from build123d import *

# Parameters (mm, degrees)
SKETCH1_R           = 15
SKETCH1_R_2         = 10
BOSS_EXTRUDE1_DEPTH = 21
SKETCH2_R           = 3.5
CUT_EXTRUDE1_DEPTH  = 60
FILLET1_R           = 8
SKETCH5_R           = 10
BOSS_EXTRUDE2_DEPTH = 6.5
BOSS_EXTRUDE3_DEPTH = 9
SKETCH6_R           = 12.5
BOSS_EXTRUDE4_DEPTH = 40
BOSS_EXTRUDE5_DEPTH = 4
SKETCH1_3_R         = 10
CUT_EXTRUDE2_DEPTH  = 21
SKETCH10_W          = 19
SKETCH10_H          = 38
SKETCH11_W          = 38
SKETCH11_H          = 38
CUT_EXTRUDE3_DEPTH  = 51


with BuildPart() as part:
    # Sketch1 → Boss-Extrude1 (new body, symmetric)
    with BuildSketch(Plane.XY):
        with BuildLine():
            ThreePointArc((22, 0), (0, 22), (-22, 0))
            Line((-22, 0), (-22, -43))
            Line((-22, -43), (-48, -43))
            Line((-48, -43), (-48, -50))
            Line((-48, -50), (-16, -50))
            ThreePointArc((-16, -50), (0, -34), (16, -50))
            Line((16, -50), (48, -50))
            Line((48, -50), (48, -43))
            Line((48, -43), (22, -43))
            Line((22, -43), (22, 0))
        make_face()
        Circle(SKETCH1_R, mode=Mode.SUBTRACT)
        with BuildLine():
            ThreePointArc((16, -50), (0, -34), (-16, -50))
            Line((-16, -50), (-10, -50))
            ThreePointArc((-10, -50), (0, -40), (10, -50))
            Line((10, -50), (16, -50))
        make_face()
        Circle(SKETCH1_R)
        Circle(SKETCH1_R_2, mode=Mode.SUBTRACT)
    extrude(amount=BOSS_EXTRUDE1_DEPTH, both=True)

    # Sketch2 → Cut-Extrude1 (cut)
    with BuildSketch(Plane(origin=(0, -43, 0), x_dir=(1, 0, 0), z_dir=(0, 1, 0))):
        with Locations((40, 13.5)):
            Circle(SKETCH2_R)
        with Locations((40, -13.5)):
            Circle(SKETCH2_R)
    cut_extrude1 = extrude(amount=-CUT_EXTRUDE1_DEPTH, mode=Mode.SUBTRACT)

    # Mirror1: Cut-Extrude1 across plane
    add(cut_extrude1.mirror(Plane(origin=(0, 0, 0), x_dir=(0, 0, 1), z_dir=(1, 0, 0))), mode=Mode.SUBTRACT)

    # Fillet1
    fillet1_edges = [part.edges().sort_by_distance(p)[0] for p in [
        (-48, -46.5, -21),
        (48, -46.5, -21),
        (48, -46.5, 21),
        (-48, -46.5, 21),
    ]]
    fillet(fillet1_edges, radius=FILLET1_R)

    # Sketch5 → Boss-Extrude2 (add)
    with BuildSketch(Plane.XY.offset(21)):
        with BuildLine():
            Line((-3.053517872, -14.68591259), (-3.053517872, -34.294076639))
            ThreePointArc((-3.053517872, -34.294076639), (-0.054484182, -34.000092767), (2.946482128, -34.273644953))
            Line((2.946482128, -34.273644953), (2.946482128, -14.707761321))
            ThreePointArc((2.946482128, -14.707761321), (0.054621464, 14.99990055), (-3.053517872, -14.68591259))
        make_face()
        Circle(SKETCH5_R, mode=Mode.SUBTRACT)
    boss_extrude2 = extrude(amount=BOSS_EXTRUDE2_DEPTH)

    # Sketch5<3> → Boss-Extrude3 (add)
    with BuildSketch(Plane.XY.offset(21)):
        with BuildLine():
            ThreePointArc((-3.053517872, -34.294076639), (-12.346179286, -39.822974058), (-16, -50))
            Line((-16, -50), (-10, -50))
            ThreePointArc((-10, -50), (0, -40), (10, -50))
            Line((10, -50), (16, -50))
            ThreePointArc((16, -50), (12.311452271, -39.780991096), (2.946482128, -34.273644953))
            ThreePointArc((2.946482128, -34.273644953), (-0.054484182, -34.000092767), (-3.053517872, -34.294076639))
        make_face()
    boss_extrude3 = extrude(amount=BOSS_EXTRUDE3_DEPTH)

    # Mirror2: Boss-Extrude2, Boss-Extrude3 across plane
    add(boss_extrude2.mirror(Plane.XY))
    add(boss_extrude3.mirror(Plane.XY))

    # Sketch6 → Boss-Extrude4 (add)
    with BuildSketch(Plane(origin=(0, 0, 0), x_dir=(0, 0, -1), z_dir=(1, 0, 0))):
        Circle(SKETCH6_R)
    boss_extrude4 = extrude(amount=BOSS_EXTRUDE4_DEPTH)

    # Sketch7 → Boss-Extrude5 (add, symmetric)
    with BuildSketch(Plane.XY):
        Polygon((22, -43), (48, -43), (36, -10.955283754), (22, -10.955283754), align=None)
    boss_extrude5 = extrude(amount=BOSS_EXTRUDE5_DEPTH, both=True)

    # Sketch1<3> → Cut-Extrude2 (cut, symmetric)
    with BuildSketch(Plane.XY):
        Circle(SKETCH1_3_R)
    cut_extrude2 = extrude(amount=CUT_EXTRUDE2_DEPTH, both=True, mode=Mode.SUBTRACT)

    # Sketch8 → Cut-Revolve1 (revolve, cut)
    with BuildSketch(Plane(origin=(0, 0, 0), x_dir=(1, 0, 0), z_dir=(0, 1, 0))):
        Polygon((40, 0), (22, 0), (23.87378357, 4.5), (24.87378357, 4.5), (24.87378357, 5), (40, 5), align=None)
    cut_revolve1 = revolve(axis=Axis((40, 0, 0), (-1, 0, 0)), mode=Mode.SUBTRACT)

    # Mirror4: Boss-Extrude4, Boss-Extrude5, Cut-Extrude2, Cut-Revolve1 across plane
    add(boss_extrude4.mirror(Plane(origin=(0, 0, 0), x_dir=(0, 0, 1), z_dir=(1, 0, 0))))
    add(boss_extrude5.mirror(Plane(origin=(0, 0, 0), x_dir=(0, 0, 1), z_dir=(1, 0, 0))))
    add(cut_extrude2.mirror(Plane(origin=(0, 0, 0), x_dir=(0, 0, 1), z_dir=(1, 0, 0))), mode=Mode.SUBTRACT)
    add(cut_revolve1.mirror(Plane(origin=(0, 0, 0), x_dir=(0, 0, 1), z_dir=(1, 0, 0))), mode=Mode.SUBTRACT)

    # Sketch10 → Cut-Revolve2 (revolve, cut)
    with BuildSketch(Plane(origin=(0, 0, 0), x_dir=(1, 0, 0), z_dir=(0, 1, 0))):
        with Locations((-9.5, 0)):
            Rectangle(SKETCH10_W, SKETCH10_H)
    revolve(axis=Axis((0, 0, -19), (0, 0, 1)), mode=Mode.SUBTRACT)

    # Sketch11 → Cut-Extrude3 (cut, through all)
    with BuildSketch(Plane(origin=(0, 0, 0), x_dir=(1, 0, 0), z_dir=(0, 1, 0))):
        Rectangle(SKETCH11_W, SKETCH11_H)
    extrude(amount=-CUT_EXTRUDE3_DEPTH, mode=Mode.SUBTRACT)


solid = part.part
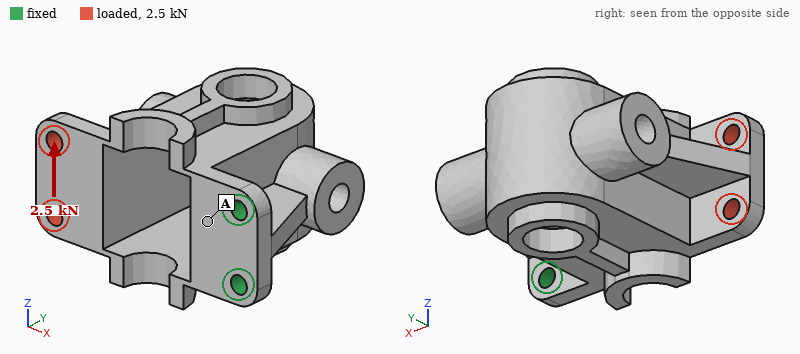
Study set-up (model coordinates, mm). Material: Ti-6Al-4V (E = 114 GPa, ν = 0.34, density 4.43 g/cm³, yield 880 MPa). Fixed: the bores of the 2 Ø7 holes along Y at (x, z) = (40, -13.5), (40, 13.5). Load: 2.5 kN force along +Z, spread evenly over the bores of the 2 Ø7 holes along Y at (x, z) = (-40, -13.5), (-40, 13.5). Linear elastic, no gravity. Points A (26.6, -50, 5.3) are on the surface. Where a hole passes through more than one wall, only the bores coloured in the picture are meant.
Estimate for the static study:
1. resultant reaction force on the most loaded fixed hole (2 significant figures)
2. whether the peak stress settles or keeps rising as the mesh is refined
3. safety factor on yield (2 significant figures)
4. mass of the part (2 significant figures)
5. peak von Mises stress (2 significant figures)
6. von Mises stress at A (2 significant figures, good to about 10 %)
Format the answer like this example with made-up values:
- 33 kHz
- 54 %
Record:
- 6.5 kN
- settles
- 1.2
- 350 g
- 730 MPa
- 72 MPa
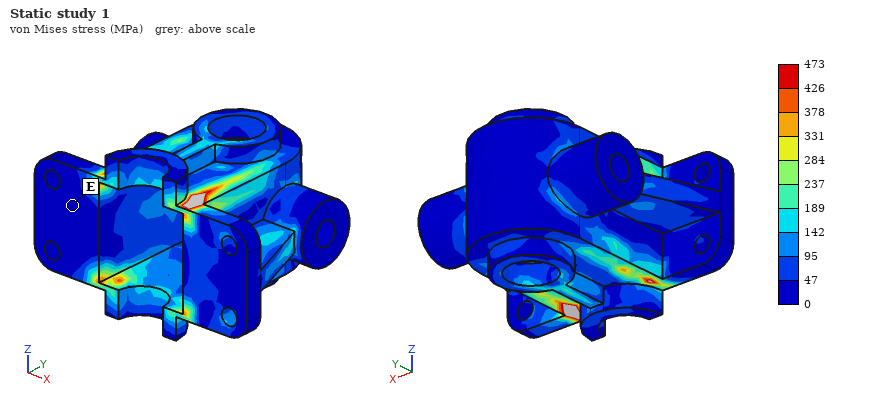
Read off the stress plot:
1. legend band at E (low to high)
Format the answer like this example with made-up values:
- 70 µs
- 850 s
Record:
- 0 to 47 MPa
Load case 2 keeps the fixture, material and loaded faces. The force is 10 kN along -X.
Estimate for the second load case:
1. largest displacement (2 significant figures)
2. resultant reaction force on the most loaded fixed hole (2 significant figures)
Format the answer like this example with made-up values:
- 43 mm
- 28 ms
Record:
- 0.21 mm
- 5.1 kN
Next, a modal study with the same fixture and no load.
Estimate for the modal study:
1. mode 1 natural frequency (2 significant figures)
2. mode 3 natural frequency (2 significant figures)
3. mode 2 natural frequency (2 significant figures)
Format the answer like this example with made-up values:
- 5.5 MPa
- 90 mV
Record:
- 690 Hz
- 1400 Hz
- 710 Hz
